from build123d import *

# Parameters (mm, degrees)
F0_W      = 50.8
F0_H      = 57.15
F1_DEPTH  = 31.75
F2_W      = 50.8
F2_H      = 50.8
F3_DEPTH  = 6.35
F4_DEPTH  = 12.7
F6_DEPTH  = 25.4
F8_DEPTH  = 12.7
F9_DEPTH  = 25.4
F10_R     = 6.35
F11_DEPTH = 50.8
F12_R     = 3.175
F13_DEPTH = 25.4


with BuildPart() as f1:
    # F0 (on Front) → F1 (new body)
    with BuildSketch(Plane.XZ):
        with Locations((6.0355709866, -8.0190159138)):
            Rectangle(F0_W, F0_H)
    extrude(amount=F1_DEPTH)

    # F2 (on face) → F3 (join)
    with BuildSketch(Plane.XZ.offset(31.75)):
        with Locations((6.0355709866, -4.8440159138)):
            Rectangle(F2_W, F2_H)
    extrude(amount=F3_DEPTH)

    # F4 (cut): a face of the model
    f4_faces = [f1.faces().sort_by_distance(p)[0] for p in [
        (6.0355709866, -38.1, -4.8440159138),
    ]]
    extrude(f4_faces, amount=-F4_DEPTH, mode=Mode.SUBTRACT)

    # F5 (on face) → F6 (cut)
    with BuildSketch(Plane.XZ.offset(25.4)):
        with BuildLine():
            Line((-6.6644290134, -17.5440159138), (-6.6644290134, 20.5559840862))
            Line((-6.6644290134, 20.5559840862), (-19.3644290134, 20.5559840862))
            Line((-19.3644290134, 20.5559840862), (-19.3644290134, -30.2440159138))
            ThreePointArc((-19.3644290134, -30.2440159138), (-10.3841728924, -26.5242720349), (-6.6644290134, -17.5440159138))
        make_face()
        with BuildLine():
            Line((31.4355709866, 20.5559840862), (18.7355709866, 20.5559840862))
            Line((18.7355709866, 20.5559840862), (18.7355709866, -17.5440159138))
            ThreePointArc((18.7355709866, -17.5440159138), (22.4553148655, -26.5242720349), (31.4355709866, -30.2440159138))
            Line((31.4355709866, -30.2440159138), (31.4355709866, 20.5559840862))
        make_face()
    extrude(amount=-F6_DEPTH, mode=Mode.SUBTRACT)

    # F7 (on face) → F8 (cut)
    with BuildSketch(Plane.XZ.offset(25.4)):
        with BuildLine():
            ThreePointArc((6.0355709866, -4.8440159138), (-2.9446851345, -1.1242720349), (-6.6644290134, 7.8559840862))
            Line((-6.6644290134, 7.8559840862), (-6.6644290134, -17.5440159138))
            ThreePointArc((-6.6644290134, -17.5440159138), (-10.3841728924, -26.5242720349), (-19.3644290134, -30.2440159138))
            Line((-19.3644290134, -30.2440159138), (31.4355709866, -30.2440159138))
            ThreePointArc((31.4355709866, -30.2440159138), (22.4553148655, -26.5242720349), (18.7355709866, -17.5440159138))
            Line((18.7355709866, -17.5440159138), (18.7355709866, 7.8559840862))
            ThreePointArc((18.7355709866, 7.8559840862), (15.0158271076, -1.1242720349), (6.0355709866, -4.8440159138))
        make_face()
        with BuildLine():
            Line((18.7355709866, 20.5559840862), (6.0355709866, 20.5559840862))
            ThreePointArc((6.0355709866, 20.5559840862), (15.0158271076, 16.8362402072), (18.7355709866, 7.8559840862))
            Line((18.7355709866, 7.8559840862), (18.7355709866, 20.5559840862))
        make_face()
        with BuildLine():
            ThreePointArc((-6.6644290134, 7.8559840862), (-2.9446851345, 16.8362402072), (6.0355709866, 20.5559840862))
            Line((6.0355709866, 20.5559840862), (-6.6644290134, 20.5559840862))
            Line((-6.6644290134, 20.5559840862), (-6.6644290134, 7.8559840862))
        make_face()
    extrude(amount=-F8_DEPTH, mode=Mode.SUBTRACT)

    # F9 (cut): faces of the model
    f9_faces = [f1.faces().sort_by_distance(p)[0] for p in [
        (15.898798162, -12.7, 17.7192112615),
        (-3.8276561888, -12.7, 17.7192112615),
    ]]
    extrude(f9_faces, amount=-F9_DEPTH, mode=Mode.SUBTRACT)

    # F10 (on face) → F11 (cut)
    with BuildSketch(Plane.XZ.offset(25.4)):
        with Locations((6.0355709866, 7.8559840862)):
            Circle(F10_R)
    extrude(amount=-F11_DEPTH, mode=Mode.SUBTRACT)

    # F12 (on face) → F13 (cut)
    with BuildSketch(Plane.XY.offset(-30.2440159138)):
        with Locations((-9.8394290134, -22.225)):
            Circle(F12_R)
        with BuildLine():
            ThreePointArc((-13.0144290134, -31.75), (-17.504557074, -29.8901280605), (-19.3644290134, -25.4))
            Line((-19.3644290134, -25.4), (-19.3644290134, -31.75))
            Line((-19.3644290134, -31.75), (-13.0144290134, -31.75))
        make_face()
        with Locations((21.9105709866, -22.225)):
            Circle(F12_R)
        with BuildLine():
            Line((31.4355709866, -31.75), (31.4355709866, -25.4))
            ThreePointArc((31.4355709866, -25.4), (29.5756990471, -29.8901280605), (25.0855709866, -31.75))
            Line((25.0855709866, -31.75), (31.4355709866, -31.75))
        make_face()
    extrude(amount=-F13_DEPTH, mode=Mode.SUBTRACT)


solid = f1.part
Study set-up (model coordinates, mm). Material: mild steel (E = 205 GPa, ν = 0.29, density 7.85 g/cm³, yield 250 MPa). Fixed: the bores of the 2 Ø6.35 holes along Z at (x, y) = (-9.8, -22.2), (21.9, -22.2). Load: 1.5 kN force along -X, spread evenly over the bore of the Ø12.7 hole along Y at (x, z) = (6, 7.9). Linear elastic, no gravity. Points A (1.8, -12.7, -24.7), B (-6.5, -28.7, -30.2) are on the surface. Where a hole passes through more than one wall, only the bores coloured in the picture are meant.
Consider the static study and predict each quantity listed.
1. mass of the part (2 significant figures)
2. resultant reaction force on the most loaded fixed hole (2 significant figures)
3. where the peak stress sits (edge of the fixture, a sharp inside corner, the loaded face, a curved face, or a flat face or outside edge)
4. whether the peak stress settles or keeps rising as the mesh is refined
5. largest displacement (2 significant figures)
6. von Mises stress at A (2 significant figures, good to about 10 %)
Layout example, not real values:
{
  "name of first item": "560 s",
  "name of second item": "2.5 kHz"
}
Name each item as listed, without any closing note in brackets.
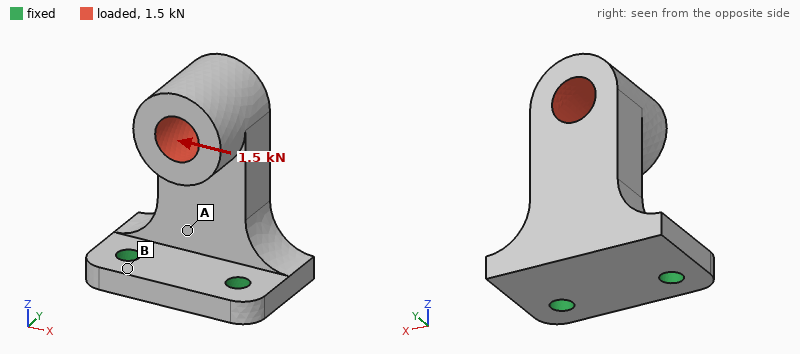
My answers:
{
  "mass of the part": "230 g",
  "resultant reaction force on the most loaded fixed hole": "2.0 kN",
  "where the peak stress sits": "edge of the fixture",
  "whether the peak stress settles or keeps rising as the mesh is refined": "keeps rising",
  "largest displacement": "49 µm",
  "von Mises stress at A": "30 MPa"
}
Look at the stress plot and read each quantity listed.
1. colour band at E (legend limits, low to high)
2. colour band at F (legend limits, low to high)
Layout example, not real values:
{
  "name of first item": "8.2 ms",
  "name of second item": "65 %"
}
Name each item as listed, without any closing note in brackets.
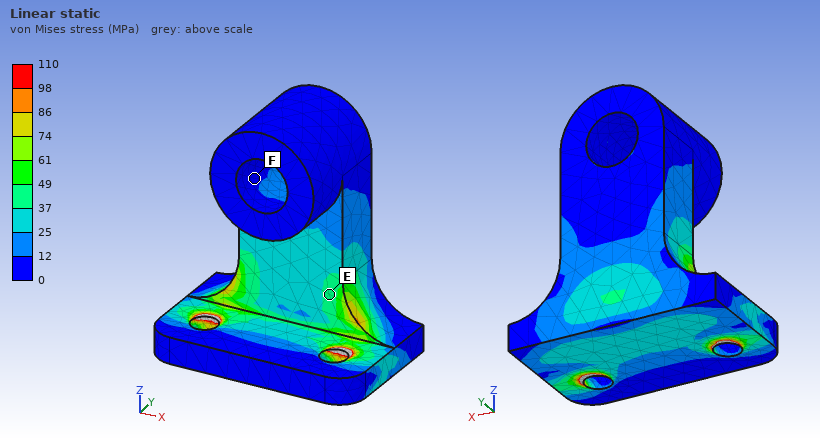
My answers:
{
  "colour band at E": "37 to 49 MPa",
  "colour band at F": "0 to 12 MPa"
}
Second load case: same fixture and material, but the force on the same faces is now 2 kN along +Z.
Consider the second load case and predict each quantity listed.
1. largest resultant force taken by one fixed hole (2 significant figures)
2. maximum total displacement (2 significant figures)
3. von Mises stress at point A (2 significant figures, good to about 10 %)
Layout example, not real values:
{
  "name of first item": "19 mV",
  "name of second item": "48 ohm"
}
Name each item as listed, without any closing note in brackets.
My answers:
{
  "largest resultant force taken by one fixed hole": "1.0 kN",
  "maximum total displacement": "11 µm",
  "von Mises stress at point A": "18 MPa"
}
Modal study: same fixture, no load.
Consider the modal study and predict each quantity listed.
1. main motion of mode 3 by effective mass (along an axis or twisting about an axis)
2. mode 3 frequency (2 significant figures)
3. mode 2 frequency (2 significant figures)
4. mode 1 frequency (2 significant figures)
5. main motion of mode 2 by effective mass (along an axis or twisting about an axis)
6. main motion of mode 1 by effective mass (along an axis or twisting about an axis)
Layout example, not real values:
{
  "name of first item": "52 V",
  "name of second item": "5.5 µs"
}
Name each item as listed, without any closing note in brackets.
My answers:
{
  "main motion of mode 3 by effective mass": "along Z",
  "mode 3 frequency": "6600 Hz",
  "mode 2 frequency": "3500 Hz",
  "mode 1 frequency": "1500 Hz",
  "main motion of mode 2 by effective mass": "along X",
  "main motion of mode 1 by effective mass": "along Y"
}
